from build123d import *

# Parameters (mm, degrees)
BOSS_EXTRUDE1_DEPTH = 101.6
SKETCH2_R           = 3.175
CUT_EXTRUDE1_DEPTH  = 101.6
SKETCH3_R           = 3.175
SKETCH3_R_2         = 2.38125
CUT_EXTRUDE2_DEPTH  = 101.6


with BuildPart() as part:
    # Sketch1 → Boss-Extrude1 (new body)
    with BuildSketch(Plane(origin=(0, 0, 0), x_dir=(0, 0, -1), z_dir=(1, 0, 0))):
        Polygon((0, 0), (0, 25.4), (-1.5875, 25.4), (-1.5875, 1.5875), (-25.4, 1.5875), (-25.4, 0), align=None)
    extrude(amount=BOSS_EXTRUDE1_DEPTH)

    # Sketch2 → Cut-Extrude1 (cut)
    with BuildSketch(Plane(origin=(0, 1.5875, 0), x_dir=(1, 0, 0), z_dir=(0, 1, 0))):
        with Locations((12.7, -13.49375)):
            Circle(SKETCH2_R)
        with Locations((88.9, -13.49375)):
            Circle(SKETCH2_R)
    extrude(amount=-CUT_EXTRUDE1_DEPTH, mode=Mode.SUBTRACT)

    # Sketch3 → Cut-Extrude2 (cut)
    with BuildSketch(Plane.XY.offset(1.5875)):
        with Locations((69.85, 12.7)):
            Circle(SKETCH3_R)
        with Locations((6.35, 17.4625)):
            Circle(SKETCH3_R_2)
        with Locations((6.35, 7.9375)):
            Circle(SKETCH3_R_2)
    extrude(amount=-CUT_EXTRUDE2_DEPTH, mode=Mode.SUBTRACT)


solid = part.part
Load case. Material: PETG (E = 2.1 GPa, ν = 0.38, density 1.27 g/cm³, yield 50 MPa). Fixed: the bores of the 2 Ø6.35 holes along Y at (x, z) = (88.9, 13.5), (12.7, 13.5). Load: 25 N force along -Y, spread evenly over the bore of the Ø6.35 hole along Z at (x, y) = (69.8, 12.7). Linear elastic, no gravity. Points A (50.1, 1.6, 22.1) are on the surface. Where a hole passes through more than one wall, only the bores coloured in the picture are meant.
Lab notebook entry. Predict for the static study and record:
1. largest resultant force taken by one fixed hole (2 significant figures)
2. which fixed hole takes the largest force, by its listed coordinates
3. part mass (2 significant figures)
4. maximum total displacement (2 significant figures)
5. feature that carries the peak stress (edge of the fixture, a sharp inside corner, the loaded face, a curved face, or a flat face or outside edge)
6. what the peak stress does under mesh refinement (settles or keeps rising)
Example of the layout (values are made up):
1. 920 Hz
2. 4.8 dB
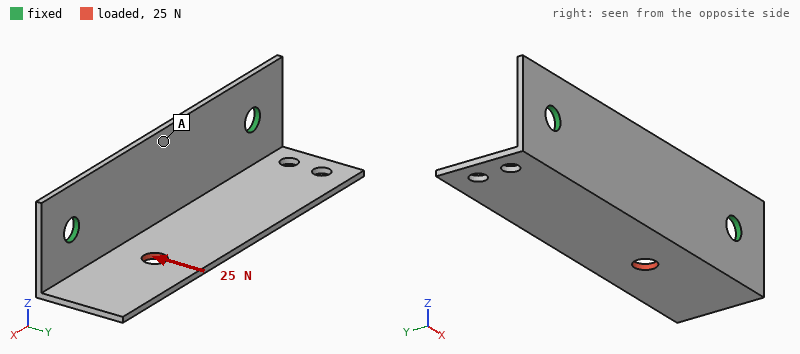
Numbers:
1. 20 N
2. (88.9, 13.5)
3. 9.8 g
4. 1.2 mm
5. edge of the fixture
6. keeps rising
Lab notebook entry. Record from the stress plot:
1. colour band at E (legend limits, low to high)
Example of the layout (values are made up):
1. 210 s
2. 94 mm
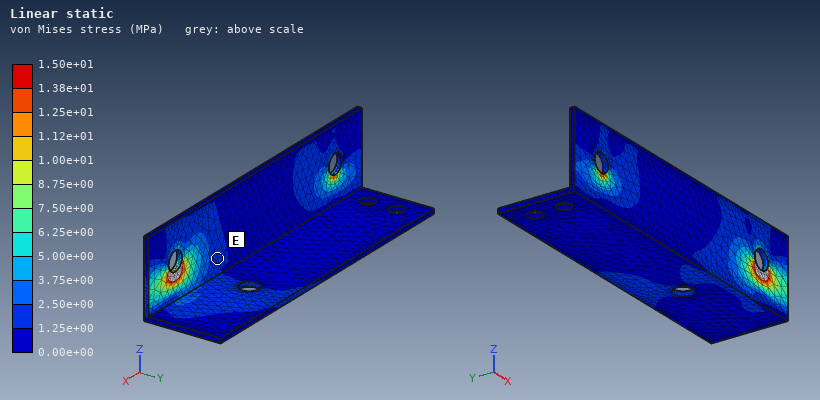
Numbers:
1. 1.25e+00 to 2.50e+00 MPa
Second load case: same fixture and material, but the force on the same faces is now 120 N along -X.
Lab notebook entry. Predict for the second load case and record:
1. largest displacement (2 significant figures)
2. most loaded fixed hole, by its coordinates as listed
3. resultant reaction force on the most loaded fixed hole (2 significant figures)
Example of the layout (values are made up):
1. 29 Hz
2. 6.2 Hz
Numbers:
1. 1.1 mm
2. (88.9, 13.5)
3. 69 N
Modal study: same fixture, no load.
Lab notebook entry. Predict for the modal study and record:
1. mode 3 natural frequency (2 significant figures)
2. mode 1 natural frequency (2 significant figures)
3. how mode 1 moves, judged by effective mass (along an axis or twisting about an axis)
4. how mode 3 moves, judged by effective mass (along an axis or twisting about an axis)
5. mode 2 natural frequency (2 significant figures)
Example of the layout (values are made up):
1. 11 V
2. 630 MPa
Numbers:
1. 560 Hz
2. 280 Hz
3. along Z
4. along Y
5. 420 Hz
